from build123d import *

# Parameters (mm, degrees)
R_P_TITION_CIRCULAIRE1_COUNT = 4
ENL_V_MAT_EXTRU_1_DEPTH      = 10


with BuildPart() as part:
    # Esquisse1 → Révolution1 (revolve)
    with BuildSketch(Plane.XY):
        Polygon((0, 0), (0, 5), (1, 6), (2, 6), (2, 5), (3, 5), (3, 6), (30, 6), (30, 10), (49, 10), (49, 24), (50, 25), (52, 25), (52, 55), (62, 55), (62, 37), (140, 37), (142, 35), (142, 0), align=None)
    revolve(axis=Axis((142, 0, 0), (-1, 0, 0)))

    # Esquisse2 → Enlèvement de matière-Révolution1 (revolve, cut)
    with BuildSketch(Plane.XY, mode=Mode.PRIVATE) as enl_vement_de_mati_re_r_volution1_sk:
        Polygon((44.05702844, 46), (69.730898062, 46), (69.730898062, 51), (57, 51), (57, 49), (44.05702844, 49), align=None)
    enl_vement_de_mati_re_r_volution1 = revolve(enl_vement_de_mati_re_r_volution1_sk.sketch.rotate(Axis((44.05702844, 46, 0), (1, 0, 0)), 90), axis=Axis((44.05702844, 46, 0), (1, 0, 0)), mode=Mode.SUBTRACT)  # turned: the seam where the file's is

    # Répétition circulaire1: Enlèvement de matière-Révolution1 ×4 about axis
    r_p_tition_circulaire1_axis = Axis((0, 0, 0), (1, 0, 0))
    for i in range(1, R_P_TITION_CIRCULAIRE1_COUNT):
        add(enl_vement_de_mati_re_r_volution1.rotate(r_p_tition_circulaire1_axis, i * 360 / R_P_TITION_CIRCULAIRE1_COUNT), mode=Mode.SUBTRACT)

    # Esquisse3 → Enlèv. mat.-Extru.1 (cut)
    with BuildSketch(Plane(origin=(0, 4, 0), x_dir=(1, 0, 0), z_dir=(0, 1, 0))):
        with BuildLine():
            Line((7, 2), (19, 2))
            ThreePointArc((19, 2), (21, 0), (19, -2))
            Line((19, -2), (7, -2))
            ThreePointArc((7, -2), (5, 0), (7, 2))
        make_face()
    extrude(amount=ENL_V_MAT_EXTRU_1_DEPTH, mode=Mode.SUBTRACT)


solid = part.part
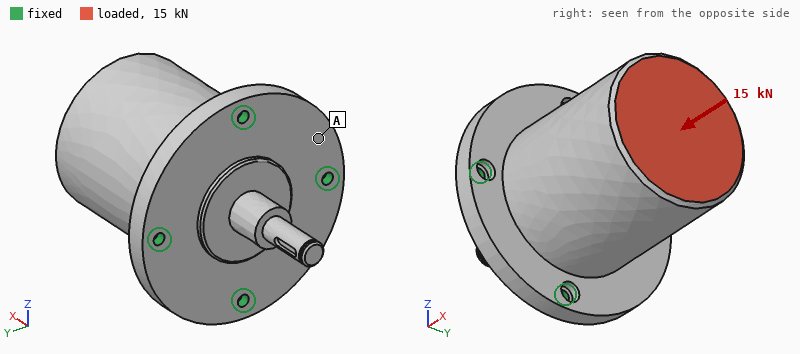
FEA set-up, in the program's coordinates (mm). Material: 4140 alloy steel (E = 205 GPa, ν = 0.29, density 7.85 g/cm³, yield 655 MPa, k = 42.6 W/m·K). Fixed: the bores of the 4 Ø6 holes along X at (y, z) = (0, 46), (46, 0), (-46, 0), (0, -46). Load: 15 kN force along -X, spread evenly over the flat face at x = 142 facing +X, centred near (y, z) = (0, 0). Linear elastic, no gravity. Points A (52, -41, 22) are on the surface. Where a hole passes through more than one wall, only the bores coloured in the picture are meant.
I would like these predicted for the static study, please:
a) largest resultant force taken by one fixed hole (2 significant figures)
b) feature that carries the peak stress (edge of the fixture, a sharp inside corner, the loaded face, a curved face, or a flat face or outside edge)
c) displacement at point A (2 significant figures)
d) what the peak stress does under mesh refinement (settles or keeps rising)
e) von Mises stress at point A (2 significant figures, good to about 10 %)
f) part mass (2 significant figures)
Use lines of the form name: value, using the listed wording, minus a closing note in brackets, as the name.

largest resultant force taken by one fixed hole: 4.3 kN
feature that carries the peak stress: edge of the fixture
displacement at point A: 5.1 µm
what the peak stress does under mesh refinement: keeps rising
von Mises stress at point A: 12 MPa
part mass: 3.5 kg
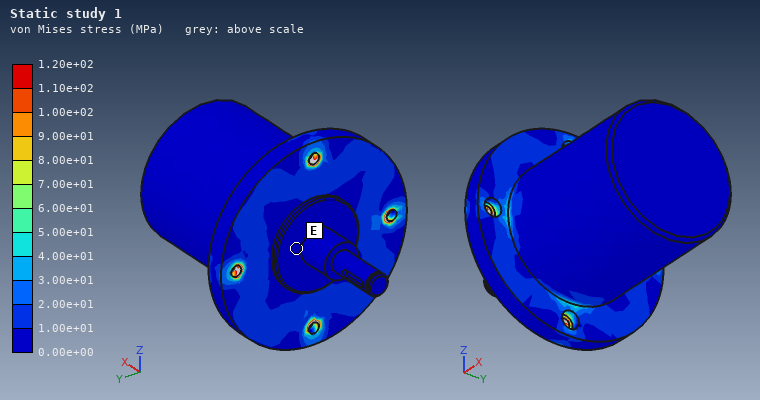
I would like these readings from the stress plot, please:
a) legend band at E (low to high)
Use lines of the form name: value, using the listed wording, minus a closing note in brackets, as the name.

legend band at E: 0.00e+00 to 1.00e+01 MPa
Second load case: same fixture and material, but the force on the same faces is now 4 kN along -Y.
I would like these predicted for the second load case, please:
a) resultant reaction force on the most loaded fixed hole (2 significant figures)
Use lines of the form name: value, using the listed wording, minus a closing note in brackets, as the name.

resultant reaction force on the most loaded fixed hole: 4.5 kN
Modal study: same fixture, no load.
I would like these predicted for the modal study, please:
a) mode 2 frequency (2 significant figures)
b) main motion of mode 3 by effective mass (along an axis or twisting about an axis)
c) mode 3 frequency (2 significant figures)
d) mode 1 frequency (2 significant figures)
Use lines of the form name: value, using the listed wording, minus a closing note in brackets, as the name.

mode 2 frequency: 2400 Hz
main motion of mode 3 by effective mass: along X
mode 3 frequency: 4100 Hz
mode 1 frequency: 2400 Hz
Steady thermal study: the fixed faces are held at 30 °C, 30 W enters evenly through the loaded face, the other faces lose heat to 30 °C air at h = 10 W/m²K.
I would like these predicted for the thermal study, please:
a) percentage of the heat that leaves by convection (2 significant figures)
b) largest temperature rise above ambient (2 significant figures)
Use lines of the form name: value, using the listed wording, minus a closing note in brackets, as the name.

percentage of the heat that leaves by convection: 15 %
largest temperature rise above ambient: 23 K
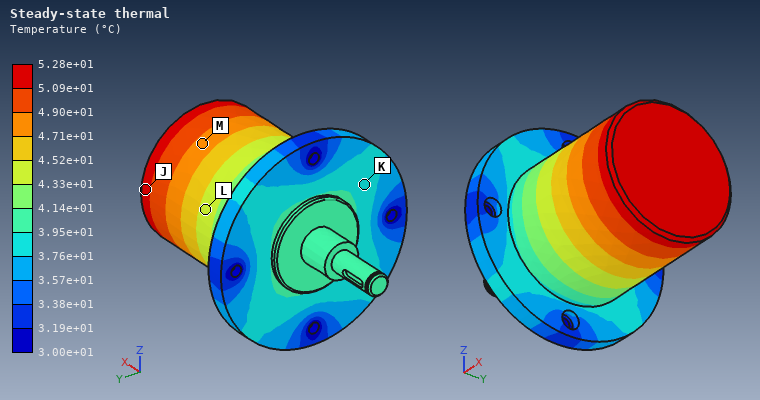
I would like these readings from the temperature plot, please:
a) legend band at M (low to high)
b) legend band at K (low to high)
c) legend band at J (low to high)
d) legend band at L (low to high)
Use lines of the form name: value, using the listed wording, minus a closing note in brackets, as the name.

legend band at M: 4.71e+01 to 4.90e+01 °C
legend band at K: 3.76e+01 to 3.95e+01 °C
legend band at J: 5.09e+01 to 5.28e+01 °C
legend band at L: 4.33e+01 to 4.52e+01 °C
